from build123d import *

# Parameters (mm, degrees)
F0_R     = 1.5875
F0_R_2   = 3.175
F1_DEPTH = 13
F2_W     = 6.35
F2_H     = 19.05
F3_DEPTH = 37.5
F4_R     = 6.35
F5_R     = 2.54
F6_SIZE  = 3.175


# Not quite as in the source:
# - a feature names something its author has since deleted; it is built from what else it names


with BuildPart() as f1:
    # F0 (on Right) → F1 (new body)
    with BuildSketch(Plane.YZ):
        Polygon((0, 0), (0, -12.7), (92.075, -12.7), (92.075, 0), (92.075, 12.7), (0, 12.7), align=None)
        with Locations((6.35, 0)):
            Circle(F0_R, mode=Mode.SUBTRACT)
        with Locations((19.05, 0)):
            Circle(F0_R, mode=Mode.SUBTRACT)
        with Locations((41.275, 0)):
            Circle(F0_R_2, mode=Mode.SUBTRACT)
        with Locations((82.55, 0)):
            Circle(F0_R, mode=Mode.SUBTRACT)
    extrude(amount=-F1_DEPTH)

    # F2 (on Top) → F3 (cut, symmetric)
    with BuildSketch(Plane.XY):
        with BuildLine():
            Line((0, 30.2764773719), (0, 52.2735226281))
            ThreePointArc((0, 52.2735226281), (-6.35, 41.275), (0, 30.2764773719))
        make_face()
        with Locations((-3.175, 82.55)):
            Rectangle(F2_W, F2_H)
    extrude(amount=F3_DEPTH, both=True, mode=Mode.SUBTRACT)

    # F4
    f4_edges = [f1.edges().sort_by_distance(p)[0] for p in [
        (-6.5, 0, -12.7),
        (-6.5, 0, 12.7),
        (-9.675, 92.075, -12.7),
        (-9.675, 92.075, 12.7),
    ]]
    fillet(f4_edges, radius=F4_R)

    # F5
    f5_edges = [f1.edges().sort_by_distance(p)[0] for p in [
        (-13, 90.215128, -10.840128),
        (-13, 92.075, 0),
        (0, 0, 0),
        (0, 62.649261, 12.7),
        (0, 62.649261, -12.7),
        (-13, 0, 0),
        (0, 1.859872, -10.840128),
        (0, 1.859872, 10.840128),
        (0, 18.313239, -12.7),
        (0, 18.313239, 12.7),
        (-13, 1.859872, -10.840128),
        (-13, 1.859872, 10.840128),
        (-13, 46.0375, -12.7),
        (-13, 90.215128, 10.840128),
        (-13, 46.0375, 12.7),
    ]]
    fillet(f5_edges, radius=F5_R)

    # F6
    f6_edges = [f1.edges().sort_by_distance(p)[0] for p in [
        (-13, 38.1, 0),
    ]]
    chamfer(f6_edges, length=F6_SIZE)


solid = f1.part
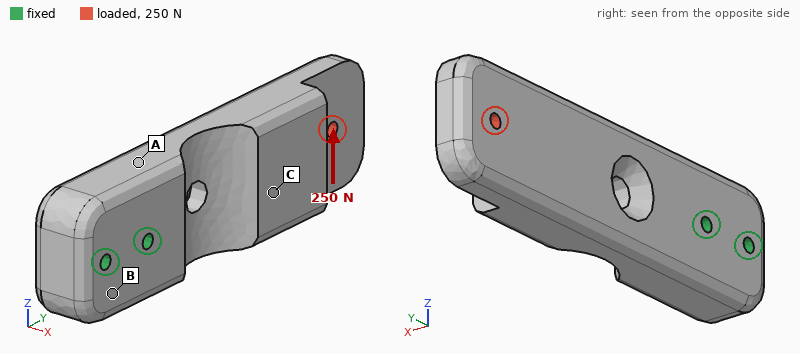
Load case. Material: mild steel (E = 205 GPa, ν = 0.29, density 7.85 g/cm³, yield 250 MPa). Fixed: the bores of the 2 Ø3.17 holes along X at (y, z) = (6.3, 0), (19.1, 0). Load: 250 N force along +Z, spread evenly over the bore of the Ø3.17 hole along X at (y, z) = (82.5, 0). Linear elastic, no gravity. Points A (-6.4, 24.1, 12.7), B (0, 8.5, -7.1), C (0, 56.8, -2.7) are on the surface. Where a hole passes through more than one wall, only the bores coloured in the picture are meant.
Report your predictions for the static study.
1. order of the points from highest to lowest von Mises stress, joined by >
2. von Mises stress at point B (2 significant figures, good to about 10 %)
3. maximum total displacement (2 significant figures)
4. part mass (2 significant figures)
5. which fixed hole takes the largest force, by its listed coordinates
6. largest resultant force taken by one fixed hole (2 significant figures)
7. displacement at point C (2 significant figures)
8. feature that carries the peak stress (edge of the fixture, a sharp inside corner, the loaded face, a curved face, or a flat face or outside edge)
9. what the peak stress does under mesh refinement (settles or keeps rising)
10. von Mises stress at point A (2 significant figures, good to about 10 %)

A > B > C
5.8 MPa
18 µm
180 g
(19.1, 0)
1.2 kN
7.2 µm
edge of the fixture
keeps rising
13 MPa
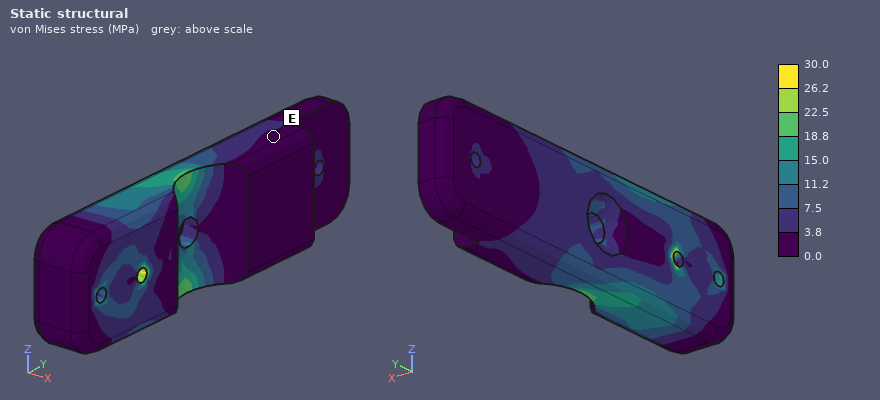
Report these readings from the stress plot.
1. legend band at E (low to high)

0.0 to 3.8 MPa
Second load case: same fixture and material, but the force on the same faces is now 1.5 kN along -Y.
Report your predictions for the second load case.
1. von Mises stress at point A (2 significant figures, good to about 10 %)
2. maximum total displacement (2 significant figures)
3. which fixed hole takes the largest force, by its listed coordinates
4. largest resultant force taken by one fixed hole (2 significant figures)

3.7 MPa
16 µm
(19.1, 0)
1.1 kN
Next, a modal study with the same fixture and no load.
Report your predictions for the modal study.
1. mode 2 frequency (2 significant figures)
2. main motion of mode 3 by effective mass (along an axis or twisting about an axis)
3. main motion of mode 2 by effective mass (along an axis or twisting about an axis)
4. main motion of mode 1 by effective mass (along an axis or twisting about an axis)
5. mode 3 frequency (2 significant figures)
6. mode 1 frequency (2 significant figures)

3000 Hz
twisting about Y
along Z
along X
6600 Hz
1300 Hz
